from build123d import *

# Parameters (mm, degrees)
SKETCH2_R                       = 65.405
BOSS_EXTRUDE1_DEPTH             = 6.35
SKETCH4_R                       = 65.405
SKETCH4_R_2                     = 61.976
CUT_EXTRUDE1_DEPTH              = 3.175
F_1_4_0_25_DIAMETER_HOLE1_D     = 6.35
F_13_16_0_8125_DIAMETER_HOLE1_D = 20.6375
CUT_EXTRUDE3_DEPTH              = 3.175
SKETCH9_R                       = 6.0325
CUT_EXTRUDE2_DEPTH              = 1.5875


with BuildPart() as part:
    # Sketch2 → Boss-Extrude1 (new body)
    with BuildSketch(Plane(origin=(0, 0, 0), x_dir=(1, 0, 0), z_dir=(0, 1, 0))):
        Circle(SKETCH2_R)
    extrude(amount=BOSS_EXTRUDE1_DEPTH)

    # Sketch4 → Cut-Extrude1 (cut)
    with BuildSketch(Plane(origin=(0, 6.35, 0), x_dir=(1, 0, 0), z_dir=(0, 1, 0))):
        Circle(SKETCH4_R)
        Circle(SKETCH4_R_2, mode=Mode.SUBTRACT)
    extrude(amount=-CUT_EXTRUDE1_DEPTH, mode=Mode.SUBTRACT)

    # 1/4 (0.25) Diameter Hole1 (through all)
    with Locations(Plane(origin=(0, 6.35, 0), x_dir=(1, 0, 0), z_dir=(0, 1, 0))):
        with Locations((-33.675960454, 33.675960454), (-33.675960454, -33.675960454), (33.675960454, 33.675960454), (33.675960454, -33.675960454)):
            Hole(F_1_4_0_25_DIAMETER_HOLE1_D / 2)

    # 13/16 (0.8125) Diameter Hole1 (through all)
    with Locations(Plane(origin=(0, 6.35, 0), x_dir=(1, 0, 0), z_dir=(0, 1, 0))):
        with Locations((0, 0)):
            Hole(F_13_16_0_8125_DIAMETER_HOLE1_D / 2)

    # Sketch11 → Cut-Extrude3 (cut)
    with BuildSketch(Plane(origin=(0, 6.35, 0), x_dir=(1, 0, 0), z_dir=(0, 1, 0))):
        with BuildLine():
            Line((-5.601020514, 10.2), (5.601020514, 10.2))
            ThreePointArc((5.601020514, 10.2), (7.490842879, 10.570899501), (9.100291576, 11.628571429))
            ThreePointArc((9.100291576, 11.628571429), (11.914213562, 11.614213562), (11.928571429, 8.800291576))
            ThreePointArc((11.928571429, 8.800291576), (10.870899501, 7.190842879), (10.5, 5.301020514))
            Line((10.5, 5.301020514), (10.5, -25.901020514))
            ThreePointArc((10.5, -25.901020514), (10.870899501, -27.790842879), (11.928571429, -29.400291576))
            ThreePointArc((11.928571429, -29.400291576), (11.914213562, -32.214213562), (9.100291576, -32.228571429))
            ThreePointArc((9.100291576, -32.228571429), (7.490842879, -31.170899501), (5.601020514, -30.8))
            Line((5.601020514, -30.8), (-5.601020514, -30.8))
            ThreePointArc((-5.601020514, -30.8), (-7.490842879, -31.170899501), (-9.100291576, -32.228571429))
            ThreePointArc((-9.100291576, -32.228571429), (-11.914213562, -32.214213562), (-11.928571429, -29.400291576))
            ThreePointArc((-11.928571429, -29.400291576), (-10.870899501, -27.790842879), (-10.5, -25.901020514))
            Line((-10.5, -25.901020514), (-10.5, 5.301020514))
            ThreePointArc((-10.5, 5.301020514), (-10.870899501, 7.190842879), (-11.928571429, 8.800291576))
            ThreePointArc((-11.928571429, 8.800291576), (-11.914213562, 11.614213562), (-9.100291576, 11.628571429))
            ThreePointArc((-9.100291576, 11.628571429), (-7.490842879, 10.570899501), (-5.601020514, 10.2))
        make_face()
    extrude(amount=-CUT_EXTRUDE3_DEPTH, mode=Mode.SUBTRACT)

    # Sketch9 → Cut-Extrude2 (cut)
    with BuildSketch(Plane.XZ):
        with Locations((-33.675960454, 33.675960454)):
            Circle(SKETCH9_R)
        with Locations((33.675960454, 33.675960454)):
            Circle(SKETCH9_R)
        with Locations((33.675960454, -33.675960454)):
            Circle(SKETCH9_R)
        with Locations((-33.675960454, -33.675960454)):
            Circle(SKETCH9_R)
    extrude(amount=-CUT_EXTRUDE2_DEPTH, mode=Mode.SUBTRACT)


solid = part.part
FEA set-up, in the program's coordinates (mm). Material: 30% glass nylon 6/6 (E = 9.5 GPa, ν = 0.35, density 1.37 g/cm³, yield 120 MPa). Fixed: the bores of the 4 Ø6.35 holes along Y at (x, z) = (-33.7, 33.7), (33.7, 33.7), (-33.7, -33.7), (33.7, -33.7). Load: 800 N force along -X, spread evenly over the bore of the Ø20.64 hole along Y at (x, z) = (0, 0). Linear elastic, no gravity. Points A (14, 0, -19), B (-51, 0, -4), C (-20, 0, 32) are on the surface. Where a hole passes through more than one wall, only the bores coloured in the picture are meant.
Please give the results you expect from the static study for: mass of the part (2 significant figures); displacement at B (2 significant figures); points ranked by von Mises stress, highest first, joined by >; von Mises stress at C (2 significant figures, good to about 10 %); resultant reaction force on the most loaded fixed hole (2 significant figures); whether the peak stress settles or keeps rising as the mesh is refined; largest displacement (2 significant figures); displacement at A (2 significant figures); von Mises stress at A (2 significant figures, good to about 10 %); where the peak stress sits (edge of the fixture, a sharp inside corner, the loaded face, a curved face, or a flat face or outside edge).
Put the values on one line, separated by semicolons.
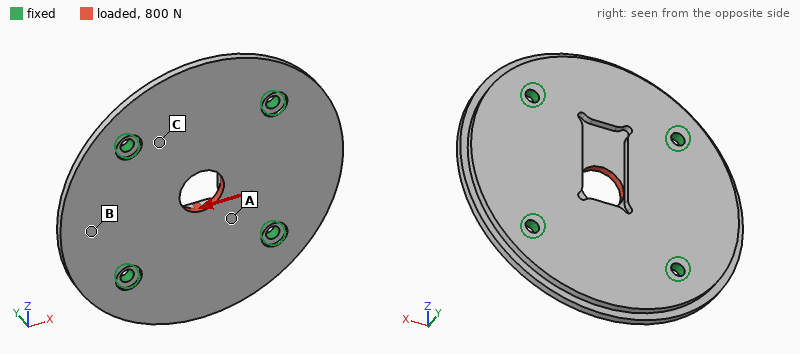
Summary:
100 g; 6.1 µm; A > C > B; 1.00 MPa; 220 N; keeps rising; 13 µm; 4.7 µm; 1.7 MPa; a sharp inside corner
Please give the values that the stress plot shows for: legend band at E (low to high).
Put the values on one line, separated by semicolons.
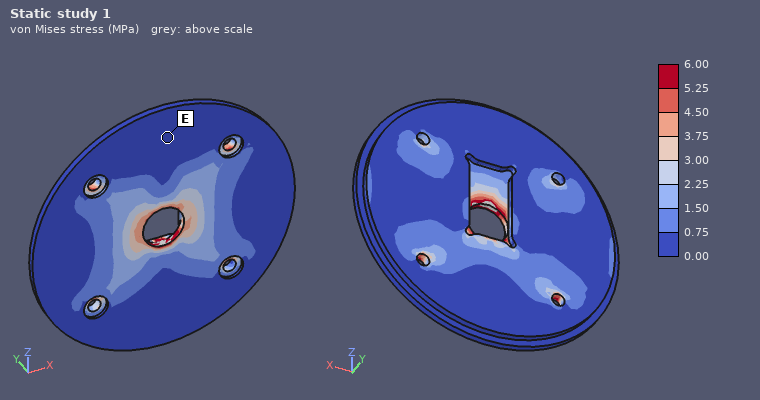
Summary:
0.00 to 0.75 MPa
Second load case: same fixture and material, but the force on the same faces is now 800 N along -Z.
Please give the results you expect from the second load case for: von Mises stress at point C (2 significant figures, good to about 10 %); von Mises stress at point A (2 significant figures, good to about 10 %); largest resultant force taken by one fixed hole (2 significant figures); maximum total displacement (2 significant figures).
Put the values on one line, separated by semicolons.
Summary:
1.1 MPa; 1.8 MPa; 210 N; 11 µm
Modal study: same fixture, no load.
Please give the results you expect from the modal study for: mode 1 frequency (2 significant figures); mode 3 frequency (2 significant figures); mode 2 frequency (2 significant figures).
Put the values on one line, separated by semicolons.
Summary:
1900 Hz; 2200 Hz; 2200 Hz
